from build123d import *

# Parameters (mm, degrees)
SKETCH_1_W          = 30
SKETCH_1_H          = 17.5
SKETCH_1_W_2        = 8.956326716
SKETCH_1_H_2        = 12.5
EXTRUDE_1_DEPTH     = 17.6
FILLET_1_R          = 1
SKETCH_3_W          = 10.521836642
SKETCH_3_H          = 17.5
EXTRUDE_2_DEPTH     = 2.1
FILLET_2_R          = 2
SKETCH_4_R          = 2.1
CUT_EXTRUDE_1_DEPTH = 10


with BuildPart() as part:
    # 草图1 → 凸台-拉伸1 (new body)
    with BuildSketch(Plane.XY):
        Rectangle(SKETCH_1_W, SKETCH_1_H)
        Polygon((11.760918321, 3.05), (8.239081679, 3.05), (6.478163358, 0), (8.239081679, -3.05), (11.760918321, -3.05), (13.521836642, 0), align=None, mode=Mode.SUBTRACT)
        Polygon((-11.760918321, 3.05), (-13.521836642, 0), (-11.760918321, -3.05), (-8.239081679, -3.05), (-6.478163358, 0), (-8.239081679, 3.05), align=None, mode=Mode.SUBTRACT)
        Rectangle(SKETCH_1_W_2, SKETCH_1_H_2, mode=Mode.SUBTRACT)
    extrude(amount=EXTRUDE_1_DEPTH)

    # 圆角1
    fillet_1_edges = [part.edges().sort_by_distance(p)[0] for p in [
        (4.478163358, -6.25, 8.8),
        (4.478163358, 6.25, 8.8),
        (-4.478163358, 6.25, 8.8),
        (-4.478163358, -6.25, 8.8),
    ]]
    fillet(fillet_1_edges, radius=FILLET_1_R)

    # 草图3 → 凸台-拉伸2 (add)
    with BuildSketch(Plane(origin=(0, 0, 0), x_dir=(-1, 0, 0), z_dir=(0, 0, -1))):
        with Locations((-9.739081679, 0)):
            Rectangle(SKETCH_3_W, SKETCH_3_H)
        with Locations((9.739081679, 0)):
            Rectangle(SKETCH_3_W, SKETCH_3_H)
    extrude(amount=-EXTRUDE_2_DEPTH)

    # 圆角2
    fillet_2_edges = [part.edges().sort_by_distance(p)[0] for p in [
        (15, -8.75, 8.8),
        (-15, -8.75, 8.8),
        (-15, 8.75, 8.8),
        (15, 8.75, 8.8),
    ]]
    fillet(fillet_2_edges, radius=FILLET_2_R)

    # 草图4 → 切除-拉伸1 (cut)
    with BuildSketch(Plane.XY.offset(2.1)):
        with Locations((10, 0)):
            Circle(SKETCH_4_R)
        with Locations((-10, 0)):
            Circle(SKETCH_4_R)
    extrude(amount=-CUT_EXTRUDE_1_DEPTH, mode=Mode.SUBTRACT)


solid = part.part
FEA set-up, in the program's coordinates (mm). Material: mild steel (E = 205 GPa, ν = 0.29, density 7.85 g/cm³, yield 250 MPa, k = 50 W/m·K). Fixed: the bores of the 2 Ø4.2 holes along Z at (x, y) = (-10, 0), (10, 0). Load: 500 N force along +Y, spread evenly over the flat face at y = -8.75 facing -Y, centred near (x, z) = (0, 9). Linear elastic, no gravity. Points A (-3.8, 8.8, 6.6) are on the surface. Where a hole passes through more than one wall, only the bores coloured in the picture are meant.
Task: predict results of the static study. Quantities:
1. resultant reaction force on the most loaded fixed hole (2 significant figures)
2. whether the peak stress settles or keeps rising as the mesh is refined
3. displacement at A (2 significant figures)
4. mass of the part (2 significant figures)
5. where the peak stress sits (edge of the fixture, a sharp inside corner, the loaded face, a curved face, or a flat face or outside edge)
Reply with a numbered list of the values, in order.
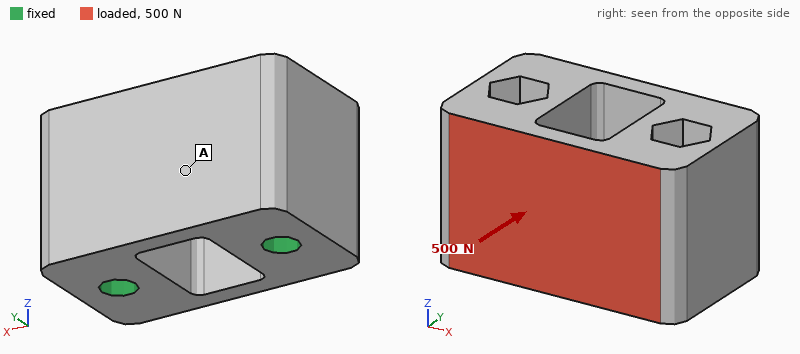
1. 250 N
2. keeps rising
3. 4.2 µm
4. 48 g
5. edge of the fixture
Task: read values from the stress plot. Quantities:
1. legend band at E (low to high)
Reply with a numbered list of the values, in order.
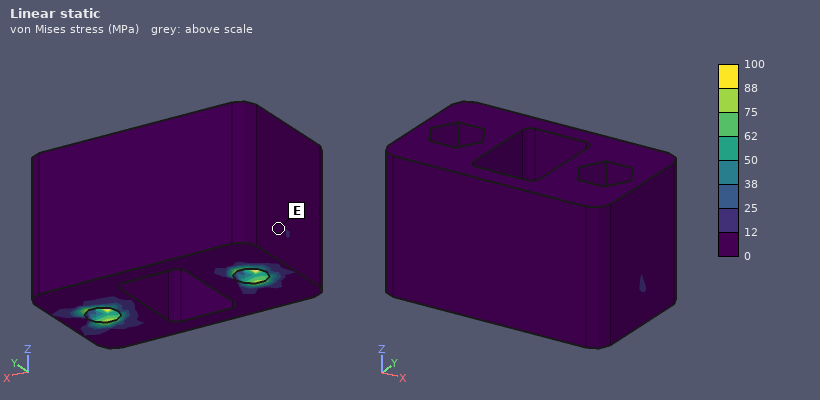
1. 0 to 12 MPa
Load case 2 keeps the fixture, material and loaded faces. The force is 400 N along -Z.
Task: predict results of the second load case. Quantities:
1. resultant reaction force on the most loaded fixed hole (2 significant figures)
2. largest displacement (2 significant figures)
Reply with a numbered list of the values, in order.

1. 200 N
2. 6.9 µm
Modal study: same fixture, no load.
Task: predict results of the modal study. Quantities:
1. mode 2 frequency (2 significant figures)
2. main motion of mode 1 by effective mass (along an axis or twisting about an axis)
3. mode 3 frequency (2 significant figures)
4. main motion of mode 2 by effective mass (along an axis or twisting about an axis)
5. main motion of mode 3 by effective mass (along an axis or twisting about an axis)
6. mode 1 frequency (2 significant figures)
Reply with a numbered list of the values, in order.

1. 18 kHz
2. along Y
3. 19 kHz
4. along X
5. twisting about Z
6. 6600 Hz
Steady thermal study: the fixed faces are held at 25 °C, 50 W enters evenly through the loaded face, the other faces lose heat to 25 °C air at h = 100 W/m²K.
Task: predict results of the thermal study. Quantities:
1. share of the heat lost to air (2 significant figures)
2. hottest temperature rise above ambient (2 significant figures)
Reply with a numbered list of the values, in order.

1. 22 %
2. 73 K
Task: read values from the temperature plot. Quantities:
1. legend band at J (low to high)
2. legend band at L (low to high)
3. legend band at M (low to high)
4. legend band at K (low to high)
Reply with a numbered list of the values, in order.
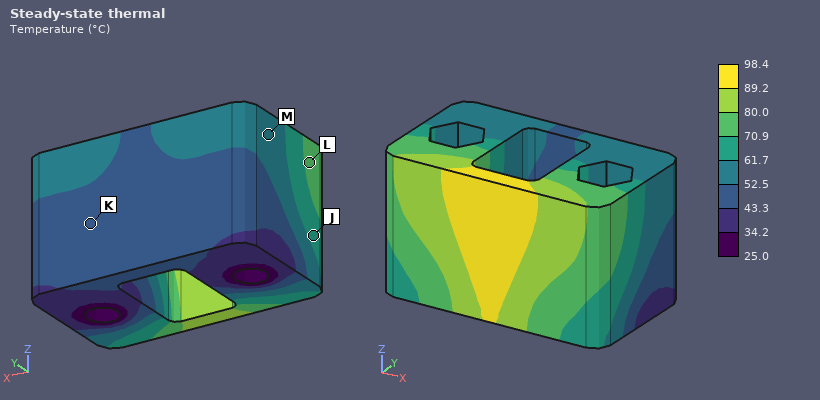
1. 61.7 to 70.9 °C
2. 70.9 to 80.0 °C
3. 52.5 to 61.7 °C
4. 43.3 to 52.5 °C
